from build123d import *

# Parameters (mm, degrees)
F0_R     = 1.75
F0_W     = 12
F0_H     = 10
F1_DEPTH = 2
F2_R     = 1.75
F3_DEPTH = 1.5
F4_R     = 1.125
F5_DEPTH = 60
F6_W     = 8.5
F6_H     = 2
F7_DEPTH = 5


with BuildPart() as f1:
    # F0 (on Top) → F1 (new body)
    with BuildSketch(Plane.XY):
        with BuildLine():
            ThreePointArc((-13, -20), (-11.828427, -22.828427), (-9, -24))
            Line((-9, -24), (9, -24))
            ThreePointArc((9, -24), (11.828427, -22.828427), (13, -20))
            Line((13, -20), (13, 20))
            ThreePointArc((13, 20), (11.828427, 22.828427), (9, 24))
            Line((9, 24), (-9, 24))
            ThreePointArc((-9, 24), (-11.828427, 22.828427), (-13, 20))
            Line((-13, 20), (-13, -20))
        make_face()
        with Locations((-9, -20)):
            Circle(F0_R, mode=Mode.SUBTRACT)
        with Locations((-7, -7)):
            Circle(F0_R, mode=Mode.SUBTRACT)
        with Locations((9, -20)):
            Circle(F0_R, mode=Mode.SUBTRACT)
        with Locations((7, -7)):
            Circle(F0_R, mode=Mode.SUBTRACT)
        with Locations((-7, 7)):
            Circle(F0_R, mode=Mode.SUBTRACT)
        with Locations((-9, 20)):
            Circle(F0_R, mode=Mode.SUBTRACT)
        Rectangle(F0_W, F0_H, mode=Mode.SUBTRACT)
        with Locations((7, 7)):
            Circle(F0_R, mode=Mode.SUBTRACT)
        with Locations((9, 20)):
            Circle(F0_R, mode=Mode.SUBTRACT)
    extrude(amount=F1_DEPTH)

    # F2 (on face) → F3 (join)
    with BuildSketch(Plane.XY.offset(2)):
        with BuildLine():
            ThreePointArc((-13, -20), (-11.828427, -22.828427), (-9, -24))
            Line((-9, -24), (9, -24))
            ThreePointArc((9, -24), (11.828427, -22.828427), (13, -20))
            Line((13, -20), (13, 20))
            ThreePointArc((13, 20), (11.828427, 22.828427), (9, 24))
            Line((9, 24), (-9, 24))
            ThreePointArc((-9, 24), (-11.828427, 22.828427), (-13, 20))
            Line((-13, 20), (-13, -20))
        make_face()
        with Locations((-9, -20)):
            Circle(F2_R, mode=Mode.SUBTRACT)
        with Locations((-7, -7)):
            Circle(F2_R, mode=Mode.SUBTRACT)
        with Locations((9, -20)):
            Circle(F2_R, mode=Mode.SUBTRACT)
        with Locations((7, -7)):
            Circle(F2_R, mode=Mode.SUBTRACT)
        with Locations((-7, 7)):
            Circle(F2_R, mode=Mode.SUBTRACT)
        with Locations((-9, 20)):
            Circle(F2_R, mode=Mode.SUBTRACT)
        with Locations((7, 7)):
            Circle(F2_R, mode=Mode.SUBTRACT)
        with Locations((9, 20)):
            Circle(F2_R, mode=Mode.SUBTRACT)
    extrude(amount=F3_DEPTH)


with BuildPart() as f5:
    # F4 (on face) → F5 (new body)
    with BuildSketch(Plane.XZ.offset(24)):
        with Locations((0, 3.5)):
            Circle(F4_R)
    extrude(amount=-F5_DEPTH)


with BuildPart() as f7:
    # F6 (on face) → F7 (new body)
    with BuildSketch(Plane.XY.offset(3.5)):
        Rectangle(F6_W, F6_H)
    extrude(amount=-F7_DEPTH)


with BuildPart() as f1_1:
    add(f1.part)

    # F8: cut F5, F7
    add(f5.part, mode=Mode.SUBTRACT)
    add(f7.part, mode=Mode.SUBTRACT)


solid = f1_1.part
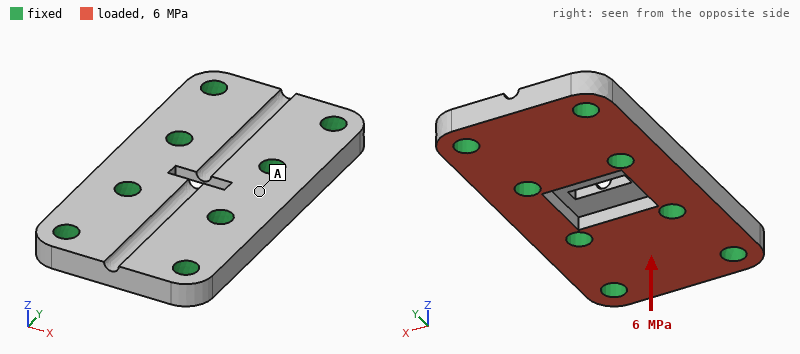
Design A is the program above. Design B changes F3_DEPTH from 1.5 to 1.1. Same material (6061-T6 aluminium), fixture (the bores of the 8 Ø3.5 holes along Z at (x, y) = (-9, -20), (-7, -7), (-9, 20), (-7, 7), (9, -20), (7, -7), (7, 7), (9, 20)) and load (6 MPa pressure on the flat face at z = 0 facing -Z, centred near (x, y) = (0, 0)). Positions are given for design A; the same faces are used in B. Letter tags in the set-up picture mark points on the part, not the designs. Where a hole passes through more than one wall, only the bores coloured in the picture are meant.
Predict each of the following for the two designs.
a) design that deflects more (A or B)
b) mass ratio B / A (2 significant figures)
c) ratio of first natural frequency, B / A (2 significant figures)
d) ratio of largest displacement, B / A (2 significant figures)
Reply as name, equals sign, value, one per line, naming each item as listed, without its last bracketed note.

design that deflects more = B
mass ratio B / A = 0.89
ratio of first natural frequency, B / A = 0.95
ratio of largest displacement, B / A = 1.2
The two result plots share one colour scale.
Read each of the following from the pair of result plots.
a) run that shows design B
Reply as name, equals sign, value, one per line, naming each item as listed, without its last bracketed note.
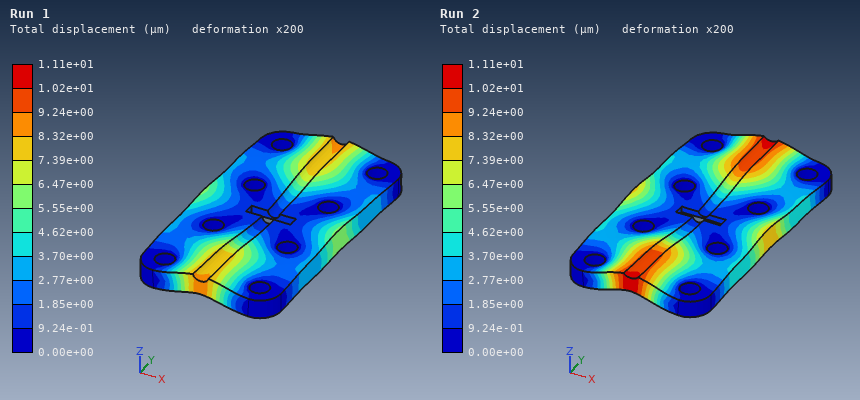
run that shows design B = Run 2
